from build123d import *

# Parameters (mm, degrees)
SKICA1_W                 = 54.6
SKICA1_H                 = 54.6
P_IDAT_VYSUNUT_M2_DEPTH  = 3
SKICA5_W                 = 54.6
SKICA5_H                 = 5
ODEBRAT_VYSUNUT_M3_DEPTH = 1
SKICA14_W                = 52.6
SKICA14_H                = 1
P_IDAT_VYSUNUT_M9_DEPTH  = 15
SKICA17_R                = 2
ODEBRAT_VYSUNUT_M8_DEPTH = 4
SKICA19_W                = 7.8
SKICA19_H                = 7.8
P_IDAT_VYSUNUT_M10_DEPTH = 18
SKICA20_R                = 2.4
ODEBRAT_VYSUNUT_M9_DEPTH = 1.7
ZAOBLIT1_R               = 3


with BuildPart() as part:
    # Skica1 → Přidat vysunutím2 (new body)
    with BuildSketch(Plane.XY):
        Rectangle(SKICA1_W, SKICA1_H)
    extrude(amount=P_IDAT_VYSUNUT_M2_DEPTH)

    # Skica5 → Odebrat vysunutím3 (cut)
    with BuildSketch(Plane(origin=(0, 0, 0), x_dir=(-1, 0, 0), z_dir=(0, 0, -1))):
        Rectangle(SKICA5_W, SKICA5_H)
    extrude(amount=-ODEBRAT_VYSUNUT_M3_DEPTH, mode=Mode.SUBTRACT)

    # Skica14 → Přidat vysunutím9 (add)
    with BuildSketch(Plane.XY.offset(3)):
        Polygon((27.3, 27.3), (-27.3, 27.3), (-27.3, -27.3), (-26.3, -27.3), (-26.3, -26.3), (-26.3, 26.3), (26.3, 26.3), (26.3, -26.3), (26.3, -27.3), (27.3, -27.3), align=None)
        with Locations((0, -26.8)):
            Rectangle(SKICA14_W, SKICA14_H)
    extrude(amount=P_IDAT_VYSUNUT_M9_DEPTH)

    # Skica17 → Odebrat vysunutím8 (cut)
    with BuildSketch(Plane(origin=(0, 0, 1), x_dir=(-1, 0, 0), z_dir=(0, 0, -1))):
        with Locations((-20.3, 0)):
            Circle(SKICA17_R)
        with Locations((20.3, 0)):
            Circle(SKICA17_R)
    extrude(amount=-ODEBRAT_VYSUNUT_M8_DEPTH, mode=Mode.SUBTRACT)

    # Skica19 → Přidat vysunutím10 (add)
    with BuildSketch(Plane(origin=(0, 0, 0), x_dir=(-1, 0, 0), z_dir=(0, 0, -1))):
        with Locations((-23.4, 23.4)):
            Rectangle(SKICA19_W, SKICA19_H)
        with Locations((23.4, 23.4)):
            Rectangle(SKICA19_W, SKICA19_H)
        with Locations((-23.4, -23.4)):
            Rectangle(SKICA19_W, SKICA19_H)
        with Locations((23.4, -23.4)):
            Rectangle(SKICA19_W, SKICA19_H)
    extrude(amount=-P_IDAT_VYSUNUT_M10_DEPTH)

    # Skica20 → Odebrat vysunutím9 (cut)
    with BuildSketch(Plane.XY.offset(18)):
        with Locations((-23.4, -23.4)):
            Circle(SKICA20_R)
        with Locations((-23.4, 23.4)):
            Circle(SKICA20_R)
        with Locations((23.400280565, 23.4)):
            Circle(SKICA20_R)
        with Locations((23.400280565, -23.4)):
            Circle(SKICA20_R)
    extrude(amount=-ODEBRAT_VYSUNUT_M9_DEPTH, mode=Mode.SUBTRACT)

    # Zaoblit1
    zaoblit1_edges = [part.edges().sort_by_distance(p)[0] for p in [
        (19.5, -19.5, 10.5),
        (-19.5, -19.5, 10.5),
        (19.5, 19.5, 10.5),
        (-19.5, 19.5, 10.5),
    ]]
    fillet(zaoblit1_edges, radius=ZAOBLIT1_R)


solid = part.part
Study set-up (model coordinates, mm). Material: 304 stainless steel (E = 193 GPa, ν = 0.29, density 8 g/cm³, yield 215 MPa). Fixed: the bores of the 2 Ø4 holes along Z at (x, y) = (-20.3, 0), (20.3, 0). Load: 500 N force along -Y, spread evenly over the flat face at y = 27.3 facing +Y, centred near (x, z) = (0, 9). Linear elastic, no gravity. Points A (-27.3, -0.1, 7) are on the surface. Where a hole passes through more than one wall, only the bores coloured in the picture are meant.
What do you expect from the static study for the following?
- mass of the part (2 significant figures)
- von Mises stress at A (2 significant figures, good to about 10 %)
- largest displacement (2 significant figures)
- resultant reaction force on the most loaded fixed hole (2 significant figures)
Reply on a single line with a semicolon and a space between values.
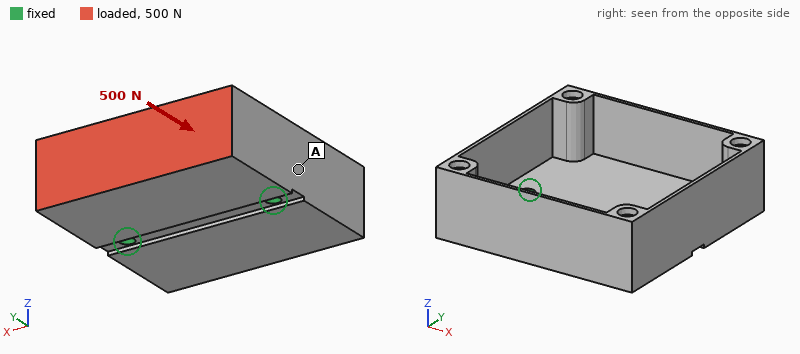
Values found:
110 g; 17 MPa; 0.12 mm; 250 N
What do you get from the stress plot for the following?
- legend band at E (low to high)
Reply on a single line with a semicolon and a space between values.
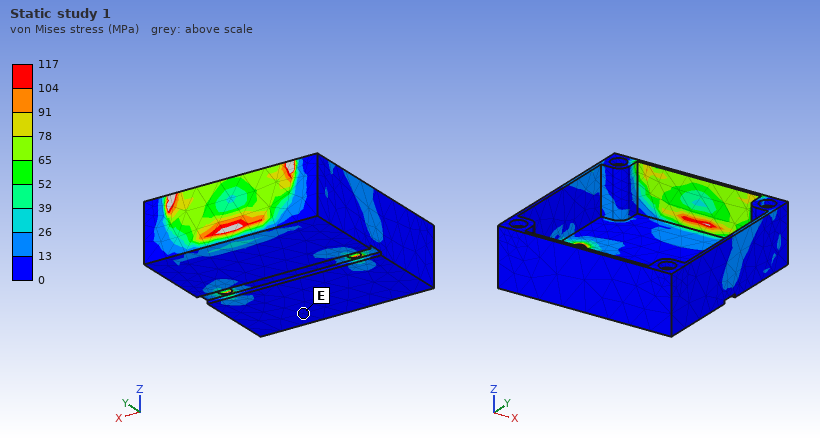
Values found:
0 to 13 MPa
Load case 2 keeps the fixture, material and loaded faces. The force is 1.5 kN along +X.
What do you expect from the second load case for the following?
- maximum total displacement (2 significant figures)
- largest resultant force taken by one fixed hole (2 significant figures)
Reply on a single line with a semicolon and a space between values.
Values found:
96 µm; 1.2 kN
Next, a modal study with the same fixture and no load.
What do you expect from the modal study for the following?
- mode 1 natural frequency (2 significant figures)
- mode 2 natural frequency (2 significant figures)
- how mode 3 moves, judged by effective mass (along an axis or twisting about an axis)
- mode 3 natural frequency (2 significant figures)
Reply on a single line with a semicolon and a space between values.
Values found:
1500 Hz; 2200 Hz; along Z; 4400 Hz
